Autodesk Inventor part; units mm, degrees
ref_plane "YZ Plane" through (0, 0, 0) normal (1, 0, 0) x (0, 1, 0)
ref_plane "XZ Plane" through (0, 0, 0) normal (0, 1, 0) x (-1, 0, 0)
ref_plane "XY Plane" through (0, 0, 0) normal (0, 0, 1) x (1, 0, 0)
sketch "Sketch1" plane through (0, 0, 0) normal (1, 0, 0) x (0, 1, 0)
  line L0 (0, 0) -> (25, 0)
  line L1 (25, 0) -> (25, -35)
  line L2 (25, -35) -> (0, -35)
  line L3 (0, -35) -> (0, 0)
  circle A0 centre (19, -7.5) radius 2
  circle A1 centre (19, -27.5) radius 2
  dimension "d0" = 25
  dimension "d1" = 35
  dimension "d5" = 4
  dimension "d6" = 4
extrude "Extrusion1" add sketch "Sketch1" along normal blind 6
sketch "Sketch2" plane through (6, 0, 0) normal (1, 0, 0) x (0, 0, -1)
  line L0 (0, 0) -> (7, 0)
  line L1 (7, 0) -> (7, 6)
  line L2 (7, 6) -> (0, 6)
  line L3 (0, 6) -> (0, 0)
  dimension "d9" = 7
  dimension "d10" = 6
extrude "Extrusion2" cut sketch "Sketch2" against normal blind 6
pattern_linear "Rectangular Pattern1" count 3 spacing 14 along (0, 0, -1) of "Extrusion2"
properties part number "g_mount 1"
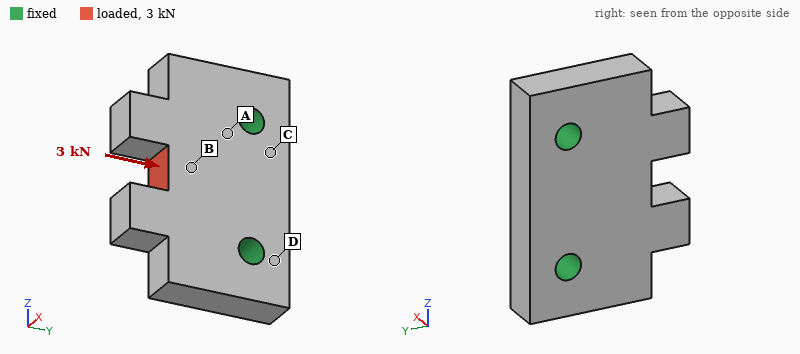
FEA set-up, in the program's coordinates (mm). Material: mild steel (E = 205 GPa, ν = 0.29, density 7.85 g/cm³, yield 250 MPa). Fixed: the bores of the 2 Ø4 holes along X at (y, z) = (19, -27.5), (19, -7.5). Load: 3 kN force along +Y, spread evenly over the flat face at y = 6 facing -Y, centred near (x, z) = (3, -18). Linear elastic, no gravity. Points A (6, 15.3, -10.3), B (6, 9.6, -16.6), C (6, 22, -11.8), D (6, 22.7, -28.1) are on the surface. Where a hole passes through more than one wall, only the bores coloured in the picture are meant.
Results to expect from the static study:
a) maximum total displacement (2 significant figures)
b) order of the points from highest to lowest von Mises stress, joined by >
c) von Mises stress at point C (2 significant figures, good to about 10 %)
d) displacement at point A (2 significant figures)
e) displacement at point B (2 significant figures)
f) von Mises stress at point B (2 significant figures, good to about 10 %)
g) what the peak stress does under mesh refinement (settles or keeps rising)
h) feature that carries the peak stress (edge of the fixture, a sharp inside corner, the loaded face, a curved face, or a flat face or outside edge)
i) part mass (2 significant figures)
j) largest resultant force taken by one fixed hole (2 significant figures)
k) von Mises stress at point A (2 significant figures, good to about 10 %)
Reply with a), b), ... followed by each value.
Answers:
a) 3.8 µm
b) B > A > C > D
c) 19 MPa
d) 0.64 µm
e) 2.6 µm
f) 53 MPa
g) keeps rising
h) edge of the fixture
i) 34 g
j) 1.6 kN
k) 38 MPa
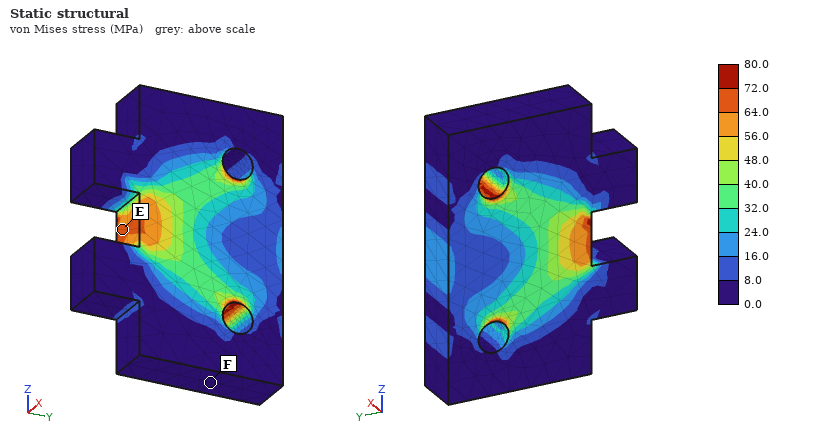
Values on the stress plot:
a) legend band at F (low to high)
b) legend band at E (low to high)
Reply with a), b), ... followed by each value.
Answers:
a) 0.0 to 8.0 MPa
b) 64.0 to 72.0 MPa
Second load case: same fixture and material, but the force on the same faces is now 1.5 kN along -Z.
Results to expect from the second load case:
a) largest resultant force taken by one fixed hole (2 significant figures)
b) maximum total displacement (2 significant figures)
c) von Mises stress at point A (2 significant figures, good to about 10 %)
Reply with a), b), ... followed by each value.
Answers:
a) 1.1 kN
b) 2.6 µm
c) 22 MPa
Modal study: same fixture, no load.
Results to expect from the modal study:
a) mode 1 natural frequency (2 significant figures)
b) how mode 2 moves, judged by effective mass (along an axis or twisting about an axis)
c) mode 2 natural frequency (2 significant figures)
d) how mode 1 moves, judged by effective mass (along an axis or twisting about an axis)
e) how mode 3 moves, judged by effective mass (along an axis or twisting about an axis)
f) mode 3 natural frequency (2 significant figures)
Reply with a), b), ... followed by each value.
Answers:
a) 16 kHz
b) twisting about Y
c) 23 kHz
d) along X
e) along Z
f) 37 kHz
